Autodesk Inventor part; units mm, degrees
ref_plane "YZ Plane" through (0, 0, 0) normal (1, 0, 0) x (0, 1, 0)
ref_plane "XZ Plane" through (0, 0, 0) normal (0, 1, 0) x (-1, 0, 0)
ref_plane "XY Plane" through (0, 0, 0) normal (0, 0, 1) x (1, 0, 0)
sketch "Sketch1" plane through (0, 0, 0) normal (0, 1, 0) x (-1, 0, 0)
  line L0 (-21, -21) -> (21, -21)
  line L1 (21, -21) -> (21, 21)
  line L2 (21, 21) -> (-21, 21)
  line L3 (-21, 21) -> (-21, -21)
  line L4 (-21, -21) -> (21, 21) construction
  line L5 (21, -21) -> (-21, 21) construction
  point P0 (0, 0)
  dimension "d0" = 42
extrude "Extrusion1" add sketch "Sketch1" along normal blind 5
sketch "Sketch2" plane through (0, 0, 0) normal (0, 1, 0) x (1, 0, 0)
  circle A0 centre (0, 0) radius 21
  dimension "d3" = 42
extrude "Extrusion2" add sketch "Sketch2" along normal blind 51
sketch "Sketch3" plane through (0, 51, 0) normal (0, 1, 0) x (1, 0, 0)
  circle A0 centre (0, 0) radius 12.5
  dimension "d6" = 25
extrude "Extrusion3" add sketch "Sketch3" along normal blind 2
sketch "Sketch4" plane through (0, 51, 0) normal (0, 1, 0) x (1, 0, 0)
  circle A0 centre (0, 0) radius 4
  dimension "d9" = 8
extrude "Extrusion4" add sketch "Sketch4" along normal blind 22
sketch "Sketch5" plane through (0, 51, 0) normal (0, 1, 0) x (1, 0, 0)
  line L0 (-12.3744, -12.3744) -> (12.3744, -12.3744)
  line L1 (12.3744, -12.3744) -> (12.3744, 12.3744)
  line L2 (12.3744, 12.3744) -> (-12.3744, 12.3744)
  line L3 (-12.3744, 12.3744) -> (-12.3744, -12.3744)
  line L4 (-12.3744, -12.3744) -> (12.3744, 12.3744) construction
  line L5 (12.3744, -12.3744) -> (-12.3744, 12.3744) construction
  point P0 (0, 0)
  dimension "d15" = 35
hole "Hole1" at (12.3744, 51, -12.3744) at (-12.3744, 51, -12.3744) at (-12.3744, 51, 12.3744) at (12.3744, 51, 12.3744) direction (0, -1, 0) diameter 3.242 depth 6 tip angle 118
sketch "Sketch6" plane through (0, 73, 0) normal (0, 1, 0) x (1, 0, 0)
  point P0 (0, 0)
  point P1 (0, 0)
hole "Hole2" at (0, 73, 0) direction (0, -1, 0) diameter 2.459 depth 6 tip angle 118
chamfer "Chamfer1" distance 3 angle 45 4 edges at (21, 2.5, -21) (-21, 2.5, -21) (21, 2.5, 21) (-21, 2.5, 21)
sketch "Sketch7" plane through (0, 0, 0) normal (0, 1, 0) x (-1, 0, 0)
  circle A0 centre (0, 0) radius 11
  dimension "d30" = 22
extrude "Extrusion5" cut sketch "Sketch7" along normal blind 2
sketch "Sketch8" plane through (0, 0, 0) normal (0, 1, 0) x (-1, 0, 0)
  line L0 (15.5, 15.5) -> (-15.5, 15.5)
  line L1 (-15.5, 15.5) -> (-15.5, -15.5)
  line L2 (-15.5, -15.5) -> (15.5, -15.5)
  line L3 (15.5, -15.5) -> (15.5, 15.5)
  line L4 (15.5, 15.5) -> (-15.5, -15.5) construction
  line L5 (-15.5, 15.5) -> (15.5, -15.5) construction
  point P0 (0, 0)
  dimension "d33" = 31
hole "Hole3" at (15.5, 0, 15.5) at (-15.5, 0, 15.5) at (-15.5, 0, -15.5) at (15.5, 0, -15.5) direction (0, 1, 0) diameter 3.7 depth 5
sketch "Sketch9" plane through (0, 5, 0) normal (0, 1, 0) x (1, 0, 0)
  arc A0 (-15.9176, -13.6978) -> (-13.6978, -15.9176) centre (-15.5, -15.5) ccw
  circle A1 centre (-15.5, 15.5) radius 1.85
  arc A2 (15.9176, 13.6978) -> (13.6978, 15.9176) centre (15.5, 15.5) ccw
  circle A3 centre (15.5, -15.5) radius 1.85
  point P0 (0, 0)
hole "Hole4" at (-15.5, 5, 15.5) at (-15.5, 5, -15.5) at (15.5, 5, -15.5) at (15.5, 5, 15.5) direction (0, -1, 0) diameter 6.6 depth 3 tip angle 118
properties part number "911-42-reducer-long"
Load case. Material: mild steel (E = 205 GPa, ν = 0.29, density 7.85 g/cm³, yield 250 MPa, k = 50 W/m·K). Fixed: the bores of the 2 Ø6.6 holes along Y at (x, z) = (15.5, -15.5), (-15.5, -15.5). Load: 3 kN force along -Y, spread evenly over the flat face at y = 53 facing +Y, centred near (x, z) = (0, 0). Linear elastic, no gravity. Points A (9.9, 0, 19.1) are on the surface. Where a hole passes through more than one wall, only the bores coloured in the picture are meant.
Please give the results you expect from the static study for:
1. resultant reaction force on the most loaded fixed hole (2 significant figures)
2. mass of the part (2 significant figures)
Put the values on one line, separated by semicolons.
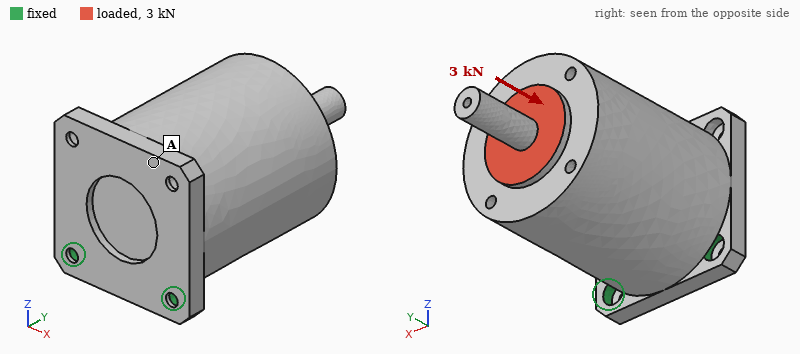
1.6 kN; 570 g
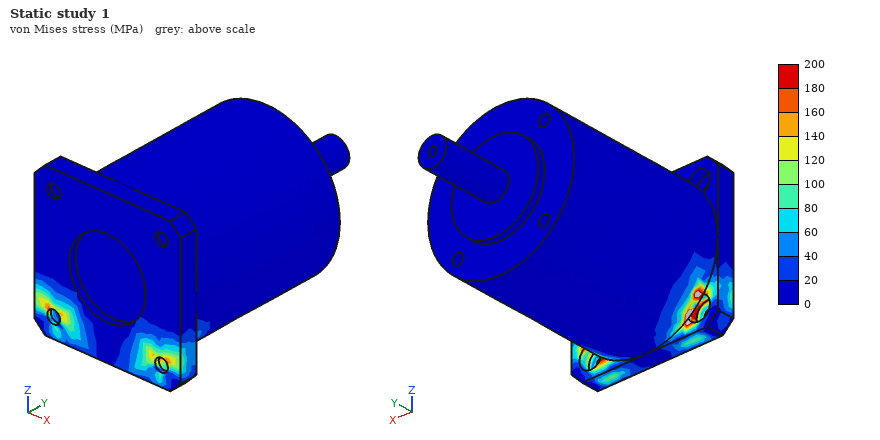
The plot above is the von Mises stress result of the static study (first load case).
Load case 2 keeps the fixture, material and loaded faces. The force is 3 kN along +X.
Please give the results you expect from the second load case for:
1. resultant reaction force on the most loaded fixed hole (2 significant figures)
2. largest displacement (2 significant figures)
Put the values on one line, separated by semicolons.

5.6 kN; 27 µm
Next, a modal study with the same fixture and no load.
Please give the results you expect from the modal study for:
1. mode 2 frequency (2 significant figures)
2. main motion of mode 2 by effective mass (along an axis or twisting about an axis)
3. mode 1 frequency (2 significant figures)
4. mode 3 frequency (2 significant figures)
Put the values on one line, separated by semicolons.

4500 Hz; along X; 1100 Hz; 8600 Hz
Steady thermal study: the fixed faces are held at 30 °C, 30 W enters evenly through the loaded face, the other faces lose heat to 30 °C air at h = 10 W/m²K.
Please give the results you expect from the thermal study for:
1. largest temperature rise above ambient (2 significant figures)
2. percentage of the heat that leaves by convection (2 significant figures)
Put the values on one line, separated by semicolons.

42 K; 8.9 %
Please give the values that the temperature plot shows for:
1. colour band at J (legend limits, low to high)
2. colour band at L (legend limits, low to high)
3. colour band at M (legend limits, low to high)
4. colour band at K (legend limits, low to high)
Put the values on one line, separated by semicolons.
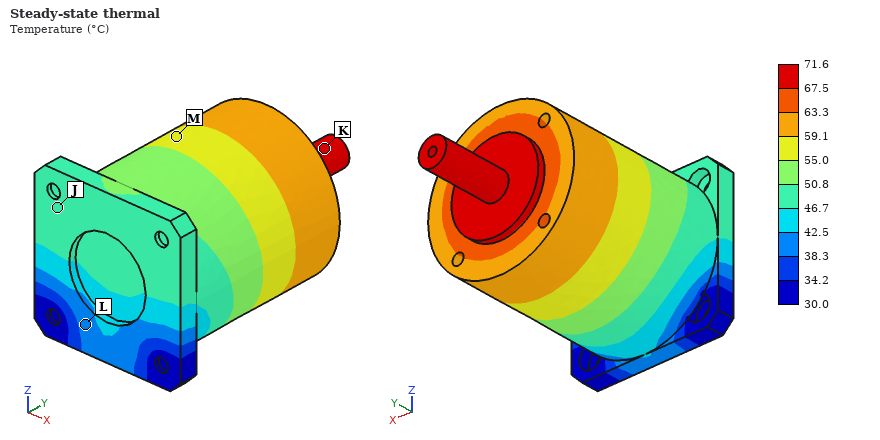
46.7 to 50.8 °C; 38.3 to 42.5 °C; 55.0 to 59.1 °C; 67.5 to 71.6 °C
